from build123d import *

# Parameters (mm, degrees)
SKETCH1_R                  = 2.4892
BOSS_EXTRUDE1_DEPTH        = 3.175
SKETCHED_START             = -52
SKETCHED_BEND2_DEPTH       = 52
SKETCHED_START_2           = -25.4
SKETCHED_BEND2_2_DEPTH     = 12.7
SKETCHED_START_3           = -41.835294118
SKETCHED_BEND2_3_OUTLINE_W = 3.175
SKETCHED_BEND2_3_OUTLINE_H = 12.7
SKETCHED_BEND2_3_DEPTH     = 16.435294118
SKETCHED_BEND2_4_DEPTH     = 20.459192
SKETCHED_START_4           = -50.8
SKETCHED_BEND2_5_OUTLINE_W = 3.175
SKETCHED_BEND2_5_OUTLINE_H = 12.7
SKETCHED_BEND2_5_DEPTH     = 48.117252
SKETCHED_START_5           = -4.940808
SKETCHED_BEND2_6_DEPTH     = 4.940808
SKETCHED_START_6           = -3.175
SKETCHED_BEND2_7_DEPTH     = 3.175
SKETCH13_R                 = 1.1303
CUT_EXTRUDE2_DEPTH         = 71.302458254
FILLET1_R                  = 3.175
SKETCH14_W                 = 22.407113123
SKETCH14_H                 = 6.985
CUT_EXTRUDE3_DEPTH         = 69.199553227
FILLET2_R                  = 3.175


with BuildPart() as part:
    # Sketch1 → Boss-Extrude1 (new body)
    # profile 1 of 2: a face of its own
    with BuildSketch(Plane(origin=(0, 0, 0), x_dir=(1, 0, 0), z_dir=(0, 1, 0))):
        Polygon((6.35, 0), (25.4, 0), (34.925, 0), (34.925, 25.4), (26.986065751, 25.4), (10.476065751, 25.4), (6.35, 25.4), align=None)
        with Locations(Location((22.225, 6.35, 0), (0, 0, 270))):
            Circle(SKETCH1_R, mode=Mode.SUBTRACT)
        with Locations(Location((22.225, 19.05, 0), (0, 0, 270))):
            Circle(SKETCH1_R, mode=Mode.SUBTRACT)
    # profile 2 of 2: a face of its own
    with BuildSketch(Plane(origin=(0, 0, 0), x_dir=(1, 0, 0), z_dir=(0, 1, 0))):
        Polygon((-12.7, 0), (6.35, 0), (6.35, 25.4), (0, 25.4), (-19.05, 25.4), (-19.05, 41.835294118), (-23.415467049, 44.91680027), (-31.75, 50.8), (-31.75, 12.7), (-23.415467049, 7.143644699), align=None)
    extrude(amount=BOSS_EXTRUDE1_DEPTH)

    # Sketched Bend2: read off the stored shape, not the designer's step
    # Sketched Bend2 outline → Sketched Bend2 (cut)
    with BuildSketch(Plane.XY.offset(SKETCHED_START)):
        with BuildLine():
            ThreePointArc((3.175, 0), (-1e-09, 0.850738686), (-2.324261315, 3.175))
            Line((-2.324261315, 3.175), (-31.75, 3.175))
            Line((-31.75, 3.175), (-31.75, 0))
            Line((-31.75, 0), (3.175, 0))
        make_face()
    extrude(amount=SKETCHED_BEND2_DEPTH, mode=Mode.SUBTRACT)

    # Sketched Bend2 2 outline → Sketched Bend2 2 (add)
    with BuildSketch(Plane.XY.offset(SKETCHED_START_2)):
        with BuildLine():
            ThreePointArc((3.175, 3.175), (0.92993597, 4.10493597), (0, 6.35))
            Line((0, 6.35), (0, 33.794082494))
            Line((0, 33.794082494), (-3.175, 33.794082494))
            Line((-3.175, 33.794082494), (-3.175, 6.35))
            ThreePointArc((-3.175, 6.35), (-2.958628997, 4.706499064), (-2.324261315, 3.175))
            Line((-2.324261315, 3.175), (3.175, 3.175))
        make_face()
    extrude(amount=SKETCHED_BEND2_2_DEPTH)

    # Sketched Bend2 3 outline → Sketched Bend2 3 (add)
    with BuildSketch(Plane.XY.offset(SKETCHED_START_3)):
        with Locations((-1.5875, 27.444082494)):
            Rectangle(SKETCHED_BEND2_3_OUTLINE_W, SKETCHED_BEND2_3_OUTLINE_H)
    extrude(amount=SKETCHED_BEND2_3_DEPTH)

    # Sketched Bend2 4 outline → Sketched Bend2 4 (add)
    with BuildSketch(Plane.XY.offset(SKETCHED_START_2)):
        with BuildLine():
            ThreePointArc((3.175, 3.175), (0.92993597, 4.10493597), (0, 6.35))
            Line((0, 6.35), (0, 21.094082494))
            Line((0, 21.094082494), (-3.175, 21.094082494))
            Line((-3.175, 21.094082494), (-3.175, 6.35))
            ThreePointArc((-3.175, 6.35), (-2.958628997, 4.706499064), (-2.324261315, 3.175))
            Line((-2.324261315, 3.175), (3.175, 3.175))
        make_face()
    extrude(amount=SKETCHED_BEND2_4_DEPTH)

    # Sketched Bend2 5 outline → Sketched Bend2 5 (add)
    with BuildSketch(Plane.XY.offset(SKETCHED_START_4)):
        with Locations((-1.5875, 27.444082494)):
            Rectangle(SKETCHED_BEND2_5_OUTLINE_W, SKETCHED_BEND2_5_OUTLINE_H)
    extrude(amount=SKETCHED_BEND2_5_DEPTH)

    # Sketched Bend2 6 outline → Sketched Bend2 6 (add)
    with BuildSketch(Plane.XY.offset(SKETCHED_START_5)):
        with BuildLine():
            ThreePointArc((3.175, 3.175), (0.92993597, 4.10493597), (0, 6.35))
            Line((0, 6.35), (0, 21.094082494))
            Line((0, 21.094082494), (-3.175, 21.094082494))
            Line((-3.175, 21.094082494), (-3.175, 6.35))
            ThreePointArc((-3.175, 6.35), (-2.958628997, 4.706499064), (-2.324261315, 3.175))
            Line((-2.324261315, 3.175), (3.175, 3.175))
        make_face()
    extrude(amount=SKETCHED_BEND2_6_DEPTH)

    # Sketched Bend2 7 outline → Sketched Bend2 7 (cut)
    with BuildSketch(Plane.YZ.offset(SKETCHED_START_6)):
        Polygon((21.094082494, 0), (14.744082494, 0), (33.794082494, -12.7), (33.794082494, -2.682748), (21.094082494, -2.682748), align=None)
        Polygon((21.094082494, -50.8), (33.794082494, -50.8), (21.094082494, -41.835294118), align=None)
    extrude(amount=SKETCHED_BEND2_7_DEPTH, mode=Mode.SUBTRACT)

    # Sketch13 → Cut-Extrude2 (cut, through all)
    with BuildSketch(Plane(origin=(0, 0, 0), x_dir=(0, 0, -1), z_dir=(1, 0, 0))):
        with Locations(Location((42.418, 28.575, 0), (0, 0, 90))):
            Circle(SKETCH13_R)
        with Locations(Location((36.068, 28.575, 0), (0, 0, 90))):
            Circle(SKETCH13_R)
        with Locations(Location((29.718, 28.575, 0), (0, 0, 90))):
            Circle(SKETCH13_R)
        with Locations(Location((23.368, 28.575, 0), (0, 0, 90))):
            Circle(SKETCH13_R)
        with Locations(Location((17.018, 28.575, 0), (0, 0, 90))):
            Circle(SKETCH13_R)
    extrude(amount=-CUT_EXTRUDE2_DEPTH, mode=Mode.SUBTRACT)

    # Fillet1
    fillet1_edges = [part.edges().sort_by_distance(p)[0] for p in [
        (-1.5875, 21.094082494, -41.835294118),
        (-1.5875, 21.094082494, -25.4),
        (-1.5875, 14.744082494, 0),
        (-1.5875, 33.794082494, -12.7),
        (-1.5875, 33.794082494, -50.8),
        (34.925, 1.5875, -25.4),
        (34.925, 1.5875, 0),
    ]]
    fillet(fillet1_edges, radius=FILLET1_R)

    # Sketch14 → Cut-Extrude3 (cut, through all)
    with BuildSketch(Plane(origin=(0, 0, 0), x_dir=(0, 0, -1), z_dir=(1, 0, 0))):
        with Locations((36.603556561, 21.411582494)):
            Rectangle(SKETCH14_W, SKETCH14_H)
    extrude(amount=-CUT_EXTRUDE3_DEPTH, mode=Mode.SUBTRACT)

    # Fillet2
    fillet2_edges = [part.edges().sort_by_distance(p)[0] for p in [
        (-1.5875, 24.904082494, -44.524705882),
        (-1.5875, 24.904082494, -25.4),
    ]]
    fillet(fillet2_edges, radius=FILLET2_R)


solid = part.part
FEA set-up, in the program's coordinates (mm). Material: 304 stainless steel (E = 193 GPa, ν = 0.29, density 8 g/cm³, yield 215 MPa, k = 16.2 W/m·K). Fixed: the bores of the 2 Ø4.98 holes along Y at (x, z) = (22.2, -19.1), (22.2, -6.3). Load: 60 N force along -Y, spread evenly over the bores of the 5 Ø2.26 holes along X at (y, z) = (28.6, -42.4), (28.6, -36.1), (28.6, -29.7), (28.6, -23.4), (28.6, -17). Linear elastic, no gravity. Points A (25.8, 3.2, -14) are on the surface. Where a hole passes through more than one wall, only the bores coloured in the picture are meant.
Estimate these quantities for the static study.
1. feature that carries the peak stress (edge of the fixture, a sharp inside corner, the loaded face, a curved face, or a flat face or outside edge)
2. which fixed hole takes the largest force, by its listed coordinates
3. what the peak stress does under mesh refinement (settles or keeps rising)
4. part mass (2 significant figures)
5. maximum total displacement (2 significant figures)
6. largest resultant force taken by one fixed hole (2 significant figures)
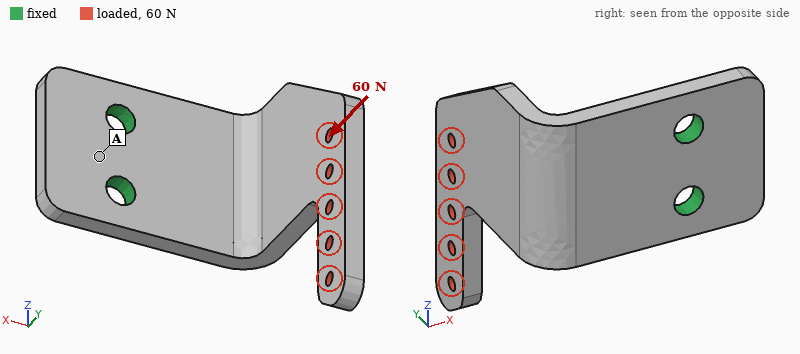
edge of the fixture
(22.2, -19.1)
keeps rising
43 g
69 µm
88 N
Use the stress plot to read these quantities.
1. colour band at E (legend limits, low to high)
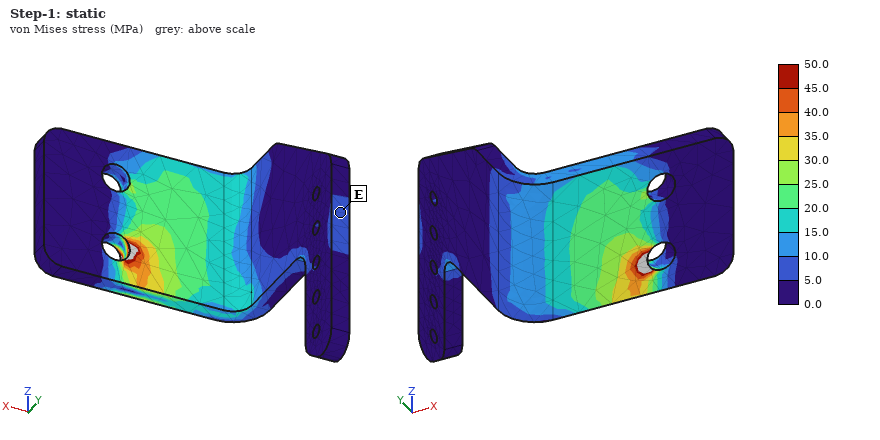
5.0 to 10.0 MPa
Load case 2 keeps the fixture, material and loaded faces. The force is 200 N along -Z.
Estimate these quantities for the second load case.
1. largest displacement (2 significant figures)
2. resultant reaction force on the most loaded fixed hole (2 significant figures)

0.19 mm
430 N
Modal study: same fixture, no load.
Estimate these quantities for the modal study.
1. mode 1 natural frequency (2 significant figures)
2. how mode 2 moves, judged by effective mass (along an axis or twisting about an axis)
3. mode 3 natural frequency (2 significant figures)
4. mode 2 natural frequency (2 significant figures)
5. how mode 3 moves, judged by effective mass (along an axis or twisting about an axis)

1000 Hz
along Z
2500 Hz
1700 Hz
along Y
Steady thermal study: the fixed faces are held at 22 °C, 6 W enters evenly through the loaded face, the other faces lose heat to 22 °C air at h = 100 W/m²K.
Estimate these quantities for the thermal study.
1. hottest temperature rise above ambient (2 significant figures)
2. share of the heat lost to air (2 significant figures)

65 K
96 %
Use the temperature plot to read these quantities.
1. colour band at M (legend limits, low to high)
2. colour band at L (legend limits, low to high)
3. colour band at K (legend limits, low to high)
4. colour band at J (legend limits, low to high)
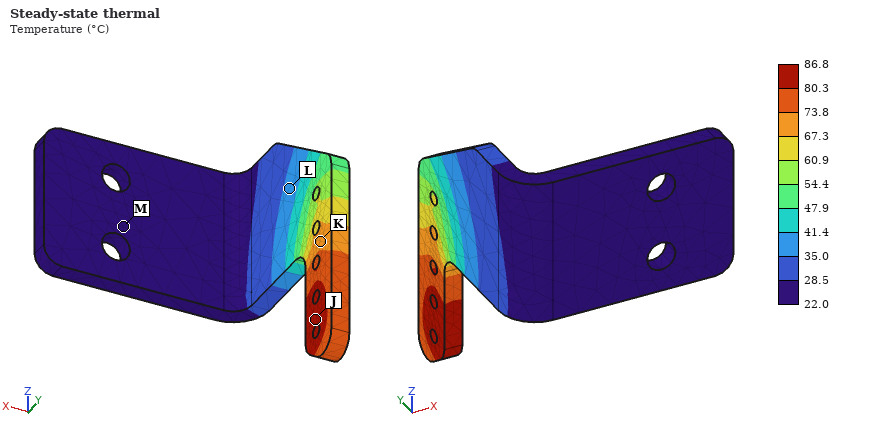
22.0 to 28.5 °C
35.0 to 41.4 °C
67.3 to 73.8 °C
80.3 to 86.8 °C
